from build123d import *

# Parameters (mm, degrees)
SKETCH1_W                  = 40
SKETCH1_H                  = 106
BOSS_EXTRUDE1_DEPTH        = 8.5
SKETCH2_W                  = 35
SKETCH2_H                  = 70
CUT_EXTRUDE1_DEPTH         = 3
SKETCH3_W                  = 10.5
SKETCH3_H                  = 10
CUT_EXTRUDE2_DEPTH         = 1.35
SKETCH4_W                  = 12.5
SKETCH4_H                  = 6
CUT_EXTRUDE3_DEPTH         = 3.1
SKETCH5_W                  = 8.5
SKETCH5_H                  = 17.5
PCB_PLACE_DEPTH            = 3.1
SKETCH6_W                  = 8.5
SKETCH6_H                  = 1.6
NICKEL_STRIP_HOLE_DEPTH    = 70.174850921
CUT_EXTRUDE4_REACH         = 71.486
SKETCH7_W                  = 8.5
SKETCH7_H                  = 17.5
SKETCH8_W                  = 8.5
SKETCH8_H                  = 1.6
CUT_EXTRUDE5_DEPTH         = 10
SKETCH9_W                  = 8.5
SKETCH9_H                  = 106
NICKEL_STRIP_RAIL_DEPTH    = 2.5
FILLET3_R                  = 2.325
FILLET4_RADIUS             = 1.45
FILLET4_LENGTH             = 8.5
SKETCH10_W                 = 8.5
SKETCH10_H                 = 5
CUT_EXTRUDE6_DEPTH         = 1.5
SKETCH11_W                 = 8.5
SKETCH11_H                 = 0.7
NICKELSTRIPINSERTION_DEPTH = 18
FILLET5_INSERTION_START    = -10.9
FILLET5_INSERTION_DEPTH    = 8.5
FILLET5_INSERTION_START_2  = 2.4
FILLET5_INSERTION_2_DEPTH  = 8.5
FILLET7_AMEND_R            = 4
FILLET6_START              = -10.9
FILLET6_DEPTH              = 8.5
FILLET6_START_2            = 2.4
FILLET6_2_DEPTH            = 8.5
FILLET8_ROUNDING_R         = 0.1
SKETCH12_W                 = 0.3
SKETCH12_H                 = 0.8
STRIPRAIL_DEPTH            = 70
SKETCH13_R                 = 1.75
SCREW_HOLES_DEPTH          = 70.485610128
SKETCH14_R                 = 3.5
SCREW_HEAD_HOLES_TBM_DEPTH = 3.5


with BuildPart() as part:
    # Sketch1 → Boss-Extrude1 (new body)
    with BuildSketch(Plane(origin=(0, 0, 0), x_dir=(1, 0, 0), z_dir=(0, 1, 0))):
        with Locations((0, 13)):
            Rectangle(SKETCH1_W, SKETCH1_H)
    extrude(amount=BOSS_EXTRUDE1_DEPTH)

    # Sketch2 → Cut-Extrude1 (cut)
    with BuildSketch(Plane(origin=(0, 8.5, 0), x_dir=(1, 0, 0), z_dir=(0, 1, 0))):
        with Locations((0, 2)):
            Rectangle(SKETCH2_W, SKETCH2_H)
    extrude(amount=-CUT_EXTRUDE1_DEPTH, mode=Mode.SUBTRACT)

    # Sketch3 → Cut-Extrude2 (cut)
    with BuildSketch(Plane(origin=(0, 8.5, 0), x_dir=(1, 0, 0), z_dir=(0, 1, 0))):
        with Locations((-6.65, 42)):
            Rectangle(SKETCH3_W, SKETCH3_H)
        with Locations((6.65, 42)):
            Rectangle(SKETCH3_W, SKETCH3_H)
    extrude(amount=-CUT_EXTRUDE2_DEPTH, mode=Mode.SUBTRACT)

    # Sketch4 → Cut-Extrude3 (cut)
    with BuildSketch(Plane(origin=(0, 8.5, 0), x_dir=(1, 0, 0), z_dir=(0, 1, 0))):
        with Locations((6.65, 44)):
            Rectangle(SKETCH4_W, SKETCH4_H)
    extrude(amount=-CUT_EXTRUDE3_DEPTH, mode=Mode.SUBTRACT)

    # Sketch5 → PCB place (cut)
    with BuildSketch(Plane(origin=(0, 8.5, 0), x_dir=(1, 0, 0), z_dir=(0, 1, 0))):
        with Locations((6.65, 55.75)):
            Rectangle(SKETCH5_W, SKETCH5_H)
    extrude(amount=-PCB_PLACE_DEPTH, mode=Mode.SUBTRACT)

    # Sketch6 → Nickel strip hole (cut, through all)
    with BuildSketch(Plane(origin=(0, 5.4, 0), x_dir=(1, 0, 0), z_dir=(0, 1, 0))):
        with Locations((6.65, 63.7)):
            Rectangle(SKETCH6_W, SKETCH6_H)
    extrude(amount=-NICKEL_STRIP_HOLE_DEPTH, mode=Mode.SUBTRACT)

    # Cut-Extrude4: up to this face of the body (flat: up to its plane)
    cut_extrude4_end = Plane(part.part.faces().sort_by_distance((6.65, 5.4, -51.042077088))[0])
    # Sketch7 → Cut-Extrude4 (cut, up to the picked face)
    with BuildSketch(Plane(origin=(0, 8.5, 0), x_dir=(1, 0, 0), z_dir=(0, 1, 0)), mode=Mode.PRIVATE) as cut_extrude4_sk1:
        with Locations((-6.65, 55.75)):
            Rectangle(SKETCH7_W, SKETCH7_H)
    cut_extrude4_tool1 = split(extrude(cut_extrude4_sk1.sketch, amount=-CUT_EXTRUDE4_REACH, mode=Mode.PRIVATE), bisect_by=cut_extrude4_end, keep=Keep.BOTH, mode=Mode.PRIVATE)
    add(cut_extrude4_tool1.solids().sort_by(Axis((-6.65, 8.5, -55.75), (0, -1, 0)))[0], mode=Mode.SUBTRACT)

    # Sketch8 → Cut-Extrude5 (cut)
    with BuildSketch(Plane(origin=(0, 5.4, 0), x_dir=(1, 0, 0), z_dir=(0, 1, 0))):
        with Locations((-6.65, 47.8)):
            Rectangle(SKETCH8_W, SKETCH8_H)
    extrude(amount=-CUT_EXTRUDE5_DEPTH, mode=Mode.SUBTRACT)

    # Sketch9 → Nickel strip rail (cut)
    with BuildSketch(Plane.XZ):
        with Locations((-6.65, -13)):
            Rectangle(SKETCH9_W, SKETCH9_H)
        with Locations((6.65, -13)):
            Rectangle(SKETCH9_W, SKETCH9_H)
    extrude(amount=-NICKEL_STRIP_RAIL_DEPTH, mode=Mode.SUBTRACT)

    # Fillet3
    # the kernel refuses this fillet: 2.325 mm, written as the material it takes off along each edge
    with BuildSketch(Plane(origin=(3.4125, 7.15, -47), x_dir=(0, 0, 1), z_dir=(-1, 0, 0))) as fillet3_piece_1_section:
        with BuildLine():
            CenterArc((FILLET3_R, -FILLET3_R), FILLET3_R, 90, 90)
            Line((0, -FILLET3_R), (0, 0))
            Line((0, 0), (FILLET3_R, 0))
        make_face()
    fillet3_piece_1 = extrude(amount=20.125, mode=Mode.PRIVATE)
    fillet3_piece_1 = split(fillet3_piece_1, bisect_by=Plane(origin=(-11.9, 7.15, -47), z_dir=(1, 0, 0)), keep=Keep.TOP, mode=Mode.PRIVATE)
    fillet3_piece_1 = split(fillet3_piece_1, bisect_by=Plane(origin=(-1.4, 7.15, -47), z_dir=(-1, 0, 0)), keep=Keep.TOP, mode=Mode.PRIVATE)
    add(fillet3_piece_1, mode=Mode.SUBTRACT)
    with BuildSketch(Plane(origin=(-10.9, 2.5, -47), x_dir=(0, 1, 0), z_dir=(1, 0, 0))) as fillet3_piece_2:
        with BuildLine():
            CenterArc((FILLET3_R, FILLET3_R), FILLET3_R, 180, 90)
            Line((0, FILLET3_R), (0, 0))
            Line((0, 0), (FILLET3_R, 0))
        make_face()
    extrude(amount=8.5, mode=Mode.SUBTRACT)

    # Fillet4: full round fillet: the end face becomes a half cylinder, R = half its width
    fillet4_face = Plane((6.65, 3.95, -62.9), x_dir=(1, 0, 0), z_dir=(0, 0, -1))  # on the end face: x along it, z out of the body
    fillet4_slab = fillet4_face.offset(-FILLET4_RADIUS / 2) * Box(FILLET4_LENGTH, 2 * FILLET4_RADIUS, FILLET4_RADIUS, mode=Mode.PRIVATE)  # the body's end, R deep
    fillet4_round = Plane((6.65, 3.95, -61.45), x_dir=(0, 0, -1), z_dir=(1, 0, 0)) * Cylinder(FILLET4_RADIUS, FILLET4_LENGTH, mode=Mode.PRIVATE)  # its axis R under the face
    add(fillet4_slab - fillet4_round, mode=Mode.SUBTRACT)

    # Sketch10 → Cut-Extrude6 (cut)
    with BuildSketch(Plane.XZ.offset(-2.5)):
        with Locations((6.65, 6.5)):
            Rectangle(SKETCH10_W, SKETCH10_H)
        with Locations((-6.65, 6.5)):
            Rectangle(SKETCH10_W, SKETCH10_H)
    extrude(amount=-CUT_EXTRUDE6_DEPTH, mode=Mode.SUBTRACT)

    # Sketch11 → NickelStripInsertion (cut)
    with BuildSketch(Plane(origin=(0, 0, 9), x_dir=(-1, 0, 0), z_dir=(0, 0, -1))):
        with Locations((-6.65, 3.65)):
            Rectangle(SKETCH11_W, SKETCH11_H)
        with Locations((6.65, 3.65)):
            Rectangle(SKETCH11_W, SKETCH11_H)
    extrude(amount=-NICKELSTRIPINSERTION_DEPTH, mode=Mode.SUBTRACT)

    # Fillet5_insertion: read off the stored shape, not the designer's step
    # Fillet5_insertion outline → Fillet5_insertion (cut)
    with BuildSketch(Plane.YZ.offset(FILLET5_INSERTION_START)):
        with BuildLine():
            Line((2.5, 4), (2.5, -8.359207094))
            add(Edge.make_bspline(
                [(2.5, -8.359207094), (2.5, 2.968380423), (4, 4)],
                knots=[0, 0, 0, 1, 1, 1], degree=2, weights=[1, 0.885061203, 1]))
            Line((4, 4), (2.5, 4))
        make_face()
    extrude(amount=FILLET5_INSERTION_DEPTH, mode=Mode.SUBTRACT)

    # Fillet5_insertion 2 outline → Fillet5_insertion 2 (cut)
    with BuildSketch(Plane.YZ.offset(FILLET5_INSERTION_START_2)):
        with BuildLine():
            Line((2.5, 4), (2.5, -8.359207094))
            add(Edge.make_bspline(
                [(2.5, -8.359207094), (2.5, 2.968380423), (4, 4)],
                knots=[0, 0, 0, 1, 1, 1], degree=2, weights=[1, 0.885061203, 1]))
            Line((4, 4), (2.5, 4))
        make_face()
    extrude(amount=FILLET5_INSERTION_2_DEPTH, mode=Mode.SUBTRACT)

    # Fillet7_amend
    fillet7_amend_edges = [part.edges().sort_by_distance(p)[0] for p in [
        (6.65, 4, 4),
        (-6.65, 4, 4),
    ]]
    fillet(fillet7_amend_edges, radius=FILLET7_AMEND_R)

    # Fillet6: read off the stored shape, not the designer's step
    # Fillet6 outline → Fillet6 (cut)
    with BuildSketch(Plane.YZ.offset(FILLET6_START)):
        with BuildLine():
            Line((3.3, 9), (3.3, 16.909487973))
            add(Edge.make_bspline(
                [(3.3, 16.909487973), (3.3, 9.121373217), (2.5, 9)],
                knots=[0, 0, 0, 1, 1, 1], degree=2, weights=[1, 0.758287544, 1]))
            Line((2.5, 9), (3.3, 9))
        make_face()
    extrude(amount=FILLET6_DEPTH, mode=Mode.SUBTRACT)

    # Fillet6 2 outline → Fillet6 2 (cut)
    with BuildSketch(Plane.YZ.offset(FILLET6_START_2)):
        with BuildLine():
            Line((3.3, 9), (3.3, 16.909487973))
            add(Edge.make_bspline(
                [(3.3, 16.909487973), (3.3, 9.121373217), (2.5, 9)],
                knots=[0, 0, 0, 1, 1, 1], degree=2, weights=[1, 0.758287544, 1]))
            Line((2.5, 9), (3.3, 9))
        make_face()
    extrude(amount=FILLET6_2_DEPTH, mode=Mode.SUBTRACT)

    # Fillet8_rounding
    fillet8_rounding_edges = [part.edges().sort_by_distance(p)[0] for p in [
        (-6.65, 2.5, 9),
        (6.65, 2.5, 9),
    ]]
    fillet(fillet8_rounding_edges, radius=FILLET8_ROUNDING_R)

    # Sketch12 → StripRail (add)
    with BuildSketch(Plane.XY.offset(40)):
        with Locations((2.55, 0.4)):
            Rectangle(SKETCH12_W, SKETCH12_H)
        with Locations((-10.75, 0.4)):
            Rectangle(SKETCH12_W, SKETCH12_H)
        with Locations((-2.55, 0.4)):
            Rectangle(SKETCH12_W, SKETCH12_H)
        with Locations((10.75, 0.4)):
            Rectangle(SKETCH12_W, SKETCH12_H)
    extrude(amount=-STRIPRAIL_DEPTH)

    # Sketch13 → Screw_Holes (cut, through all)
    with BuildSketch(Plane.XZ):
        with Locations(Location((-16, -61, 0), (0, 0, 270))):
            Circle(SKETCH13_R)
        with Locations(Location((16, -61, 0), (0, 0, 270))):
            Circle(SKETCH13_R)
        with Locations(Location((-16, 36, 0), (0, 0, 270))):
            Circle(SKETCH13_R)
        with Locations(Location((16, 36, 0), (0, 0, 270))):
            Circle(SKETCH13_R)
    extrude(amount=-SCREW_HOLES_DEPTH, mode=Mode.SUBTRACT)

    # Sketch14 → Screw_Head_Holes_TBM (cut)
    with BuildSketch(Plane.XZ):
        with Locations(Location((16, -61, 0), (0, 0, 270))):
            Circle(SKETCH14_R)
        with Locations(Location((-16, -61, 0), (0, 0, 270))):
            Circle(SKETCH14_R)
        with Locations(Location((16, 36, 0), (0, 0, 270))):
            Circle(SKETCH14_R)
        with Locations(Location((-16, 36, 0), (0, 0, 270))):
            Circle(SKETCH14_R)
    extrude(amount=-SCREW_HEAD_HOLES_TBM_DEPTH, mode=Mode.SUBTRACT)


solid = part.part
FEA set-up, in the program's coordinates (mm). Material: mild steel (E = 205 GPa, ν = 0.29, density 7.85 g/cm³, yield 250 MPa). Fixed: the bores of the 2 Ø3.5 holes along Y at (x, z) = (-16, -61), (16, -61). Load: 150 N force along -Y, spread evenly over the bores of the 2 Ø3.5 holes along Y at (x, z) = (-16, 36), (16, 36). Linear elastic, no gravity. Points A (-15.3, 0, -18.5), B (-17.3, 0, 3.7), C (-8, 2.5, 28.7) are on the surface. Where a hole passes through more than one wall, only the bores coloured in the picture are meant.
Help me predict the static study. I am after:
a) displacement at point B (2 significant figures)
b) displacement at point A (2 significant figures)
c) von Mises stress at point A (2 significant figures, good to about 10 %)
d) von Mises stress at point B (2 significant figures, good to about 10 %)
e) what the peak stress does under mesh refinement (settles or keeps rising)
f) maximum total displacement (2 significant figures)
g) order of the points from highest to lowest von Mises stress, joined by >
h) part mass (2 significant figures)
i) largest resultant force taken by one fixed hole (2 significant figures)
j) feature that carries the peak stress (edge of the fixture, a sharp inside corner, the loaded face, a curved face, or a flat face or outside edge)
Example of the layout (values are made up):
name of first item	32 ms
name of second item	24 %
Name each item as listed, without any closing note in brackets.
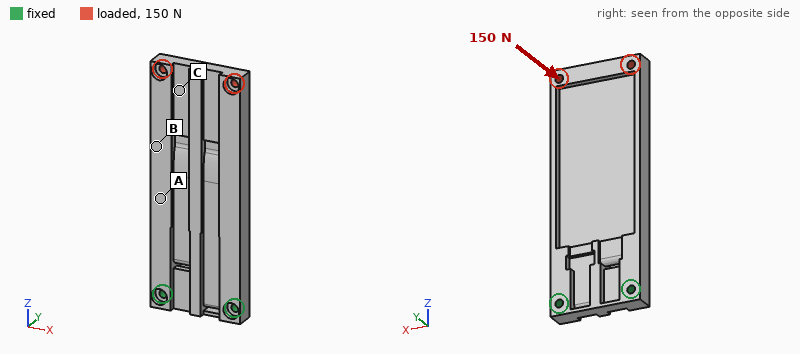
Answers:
displacement at point B	0.17 mm
displacement at point A	0.084 mm
von Mises stress at point A	43 MPa
von Mises stress at point B	26 MPa
what the peak stress does under mesh refinement	keeps rising
maximum total displacement	0.35 mm
order of the points from highest to lowest von Mises stress, joined by >	A > B > C
part mass	170 g
largest resultant force taken by one fixed hole	82 N
feature that carries the peak stress	edge of the fixture
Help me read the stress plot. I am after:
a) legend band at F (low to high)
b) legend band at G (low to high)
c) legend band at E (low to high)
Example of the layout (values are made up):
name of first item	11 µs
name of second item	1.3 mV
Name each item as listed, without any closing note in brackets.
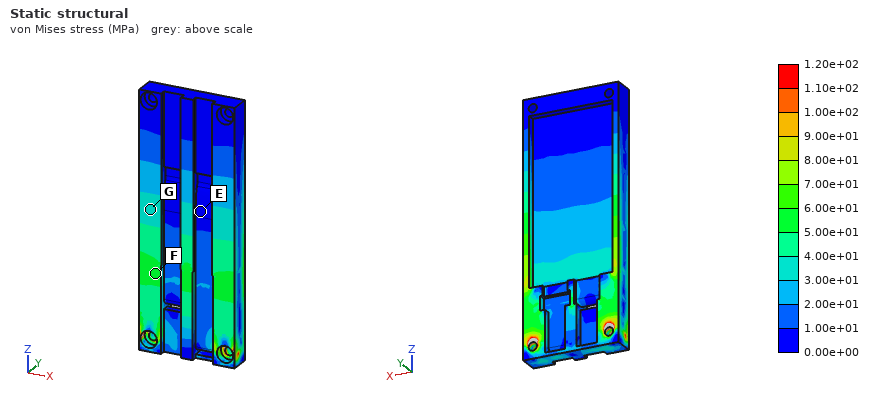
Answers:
legend band at F	5.00e+01 to 6.00e+01 MPa
legend band at G	3.00e+01 to 4.00e+01 MPa
legend band at E	0.00e+00 to 1.00e+01 MPa
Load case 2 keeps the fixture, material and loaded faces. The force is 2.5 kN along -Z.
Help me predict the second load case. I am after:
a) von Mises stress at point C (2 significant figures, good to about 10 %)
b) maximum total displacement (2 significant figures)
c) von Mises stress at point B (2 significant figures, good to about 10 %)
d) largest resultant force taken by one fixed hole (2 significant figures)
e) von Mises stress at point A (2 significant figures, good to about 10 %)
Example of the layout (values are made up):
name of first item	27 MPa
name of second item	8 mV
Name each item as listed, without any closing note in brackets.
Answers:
von Mises stress at point C	9.4 MPa
maximum total displacement	0.19 mm
von Mises stress at point B	20 MPa
largest resultant force taken by one fixed hole	1.3 kN
von Mises stress at point A	21 MPa
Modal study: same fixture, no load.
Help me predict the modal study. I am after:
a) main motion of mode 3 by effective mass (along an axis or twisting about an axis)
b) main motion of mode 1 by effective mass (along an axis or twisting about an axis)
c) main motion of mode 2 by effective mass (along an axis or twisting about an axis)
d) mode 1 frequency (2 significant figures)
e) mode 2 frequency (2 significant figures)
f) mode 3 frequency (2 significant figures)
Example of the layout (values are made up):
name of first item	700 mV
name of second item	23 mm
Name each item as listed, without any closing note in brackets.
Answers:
main motion of mode 3 by effective mass	along Y
main motion of mode 1 by effective mass	along Y
main motion of mode 2 by effective mass	twisting about Z
mode 1 frequency	510 Hz
mode 2 frequency	1800 Hz
mode 3 frequency	2900 Hz
